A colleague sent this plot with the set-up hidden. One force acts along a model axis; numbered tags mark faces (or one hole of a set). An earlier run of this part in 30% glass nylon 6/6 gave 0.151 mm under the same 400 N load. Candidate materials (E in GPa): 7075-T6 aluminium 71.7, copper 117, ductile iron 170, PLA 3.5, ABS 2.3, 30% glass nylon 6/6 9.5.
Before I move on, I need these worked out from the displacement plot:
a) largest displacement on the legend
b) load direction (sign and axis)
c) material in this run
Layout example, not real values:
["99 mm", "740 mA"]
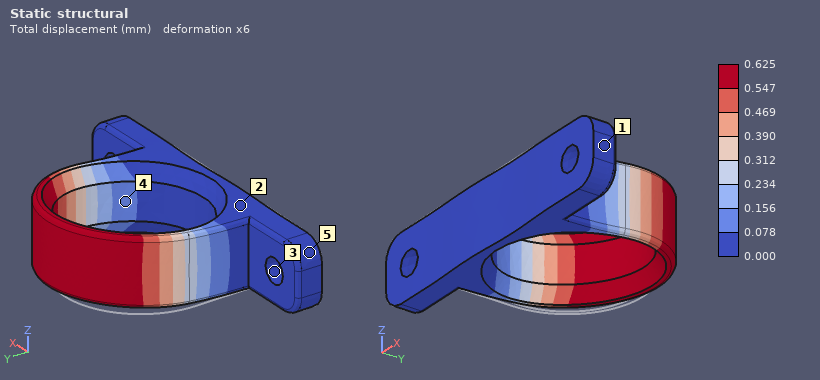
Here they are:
["0.625 mm", "+X", "ABS"]
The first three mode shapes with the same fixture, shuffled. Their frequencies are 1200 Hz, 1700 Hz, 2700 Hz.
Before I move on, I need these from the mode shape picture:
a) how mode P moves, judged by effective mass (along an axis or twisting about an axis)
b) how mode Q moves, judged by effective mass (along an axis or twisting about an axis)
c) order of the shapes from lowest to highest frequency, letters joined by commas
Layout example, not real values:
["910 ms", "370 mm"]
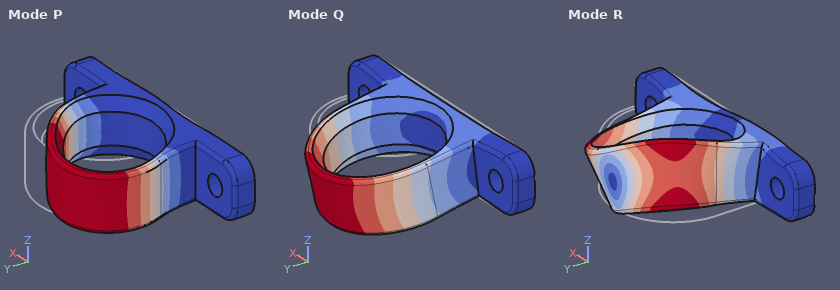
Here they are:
["along X", "along Z", "Q, P, R"]
